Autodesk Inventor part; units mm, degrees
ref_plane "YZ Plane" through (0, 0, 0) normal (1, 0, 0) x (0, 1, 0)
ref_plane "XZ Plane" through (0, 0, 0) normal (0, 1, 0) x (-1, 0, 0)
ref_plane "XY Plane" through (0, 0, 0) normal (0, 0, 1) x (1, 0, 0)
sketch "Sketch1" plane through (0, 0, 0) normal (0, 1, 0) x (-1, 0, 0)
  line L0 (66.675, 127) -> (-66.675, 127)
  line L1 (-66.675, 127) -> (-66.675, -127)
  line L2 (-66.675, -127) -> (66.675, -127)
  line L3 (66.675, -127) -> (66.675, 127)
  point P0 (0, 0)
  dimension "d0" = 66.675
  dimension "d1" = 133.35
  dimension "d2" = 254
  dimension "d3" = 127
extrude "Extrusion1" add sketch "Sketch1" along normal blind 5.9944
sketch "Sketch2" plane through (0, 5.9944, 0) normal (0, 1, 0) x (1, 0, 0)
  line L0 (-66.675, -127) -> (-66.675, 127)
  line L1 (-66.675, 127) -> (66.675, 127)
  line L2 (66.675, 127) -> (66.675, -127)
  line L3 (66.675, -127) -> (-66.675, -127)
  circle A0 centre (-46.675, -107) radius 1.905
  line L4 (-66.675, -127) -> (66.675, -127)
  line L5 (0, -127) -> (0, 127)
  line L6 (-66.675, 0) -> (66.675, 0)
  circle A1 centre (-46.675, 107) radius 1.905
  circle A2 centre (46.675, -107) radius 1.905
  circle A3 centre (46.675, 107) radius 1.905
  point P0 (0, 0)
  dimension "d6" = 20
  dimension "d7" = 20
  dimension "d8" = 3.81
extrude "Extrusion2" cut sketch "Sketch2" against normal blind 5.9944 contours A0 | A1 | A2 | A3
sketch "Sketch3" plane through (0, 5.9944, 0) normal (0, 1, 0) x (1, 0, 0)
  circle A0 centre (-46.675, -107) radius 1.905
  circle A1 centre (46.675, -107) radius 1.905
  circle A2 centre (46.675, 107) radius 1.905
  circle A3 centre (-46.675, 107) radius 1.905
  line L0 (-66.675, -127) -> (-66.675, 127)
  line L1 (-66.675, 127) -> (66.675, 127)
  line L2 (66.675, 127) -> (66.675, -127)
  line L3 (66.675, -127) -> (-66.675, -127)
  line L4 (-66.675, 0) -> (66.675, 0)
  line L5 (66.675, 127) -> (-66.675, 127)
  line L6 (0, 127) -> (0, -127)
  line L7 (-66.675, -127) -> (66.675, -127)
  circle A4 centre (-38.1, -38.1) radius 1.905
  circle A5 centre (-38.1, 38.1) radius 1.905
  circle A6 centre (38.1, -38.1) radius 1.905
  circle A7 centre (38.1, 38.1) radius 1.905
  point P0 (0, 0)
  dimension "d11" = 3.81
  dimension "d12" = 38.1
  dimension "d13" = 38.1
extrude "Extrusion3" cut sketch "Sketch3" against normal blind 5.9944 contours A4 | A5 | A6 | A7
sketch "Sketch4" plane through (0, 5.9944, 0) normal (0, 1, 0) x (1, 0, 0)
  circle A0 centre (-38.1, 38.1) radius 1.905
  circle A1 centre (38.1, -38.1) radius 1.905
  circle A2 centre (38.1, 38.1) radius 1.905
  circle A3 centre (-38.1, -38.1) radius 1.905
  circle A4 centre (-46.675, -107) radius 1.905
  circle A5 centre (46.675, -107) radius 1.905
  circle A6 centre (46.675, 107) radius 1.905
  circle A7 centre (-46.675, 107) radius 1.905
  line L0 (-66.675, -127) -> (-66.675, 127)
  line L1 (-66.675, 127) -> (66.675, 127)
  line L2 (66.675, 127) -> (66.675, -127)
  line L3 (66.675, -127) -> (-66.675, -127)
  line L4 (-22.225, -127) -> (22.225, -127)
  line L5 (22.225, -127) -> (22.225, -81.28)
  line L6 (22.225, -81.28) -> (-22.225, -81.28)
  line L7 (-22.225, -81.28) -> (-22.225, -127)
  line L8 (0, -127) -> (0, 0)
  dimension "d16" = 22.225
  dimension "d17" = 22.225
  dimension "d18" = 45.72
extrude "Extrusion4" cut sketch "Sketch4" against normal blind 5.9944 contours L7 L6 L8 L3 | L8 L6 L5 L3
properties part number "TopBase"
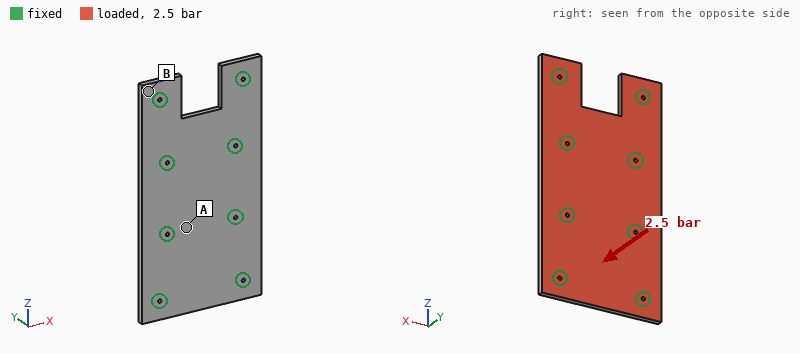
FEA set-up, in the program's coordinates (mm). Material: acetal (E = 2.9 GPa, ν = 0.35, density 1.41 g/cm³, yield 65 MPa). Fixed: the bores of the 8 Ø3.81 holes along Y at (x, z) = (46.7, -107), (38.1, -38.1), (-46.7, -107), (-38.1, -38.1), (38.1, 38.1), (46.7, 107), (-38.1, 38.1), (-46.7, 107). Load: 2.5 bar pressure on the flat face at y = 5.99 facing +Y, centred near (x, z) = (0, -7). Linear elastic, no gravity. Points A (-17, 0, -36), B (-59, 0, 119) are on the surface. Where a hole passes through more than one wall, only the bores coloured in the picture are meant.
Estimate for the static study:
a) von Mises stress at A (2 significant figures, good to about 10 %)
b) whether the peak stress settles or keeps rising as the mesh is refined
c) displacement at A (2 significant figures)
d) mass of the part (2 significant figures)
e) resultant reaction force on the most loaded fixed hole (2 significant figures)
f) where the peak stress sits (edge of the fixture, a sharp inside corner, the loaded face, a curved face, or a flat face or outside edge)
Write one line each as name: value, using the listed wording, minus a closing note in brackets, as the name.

von Mises stress at A: 12 MPa
whether the peak stress settles or keeps rising as the mesh is refined: keeps rising
displacement at A: 0.53 mm
mass of the part: 270 g
resultant reaction force on the most loaded fixed hole: 1.3 kN
where the peak stress sits: edge of the fixture
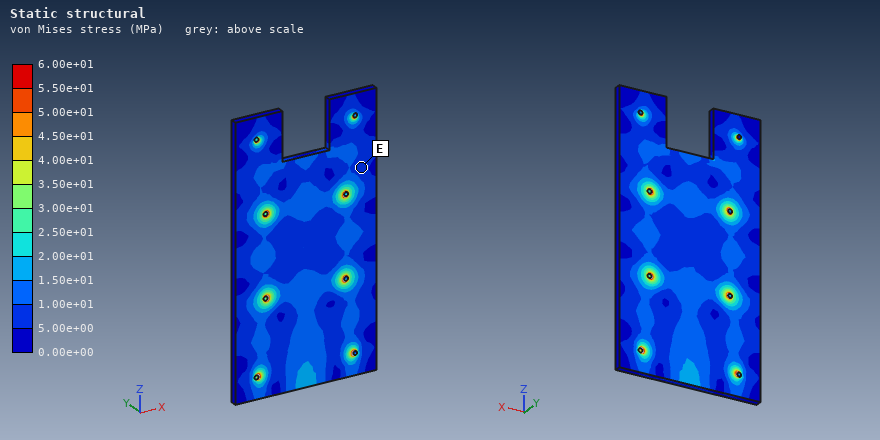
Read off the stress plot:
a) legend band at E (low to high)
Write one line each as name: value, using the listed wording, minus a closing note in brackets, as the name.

legend band at E: 5.00e+00 to 1.00e+01 MPa
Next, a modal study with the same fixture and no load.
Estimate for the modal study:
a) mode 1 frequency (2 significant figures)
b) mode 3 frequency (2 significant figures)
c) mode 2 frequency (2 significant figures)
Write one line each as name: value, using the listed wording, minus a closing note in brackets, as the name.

mode 1 frequency: 830 Hz
mode 3 frequency: 1000 Hz
mode 2 frequency: 930 Hz
